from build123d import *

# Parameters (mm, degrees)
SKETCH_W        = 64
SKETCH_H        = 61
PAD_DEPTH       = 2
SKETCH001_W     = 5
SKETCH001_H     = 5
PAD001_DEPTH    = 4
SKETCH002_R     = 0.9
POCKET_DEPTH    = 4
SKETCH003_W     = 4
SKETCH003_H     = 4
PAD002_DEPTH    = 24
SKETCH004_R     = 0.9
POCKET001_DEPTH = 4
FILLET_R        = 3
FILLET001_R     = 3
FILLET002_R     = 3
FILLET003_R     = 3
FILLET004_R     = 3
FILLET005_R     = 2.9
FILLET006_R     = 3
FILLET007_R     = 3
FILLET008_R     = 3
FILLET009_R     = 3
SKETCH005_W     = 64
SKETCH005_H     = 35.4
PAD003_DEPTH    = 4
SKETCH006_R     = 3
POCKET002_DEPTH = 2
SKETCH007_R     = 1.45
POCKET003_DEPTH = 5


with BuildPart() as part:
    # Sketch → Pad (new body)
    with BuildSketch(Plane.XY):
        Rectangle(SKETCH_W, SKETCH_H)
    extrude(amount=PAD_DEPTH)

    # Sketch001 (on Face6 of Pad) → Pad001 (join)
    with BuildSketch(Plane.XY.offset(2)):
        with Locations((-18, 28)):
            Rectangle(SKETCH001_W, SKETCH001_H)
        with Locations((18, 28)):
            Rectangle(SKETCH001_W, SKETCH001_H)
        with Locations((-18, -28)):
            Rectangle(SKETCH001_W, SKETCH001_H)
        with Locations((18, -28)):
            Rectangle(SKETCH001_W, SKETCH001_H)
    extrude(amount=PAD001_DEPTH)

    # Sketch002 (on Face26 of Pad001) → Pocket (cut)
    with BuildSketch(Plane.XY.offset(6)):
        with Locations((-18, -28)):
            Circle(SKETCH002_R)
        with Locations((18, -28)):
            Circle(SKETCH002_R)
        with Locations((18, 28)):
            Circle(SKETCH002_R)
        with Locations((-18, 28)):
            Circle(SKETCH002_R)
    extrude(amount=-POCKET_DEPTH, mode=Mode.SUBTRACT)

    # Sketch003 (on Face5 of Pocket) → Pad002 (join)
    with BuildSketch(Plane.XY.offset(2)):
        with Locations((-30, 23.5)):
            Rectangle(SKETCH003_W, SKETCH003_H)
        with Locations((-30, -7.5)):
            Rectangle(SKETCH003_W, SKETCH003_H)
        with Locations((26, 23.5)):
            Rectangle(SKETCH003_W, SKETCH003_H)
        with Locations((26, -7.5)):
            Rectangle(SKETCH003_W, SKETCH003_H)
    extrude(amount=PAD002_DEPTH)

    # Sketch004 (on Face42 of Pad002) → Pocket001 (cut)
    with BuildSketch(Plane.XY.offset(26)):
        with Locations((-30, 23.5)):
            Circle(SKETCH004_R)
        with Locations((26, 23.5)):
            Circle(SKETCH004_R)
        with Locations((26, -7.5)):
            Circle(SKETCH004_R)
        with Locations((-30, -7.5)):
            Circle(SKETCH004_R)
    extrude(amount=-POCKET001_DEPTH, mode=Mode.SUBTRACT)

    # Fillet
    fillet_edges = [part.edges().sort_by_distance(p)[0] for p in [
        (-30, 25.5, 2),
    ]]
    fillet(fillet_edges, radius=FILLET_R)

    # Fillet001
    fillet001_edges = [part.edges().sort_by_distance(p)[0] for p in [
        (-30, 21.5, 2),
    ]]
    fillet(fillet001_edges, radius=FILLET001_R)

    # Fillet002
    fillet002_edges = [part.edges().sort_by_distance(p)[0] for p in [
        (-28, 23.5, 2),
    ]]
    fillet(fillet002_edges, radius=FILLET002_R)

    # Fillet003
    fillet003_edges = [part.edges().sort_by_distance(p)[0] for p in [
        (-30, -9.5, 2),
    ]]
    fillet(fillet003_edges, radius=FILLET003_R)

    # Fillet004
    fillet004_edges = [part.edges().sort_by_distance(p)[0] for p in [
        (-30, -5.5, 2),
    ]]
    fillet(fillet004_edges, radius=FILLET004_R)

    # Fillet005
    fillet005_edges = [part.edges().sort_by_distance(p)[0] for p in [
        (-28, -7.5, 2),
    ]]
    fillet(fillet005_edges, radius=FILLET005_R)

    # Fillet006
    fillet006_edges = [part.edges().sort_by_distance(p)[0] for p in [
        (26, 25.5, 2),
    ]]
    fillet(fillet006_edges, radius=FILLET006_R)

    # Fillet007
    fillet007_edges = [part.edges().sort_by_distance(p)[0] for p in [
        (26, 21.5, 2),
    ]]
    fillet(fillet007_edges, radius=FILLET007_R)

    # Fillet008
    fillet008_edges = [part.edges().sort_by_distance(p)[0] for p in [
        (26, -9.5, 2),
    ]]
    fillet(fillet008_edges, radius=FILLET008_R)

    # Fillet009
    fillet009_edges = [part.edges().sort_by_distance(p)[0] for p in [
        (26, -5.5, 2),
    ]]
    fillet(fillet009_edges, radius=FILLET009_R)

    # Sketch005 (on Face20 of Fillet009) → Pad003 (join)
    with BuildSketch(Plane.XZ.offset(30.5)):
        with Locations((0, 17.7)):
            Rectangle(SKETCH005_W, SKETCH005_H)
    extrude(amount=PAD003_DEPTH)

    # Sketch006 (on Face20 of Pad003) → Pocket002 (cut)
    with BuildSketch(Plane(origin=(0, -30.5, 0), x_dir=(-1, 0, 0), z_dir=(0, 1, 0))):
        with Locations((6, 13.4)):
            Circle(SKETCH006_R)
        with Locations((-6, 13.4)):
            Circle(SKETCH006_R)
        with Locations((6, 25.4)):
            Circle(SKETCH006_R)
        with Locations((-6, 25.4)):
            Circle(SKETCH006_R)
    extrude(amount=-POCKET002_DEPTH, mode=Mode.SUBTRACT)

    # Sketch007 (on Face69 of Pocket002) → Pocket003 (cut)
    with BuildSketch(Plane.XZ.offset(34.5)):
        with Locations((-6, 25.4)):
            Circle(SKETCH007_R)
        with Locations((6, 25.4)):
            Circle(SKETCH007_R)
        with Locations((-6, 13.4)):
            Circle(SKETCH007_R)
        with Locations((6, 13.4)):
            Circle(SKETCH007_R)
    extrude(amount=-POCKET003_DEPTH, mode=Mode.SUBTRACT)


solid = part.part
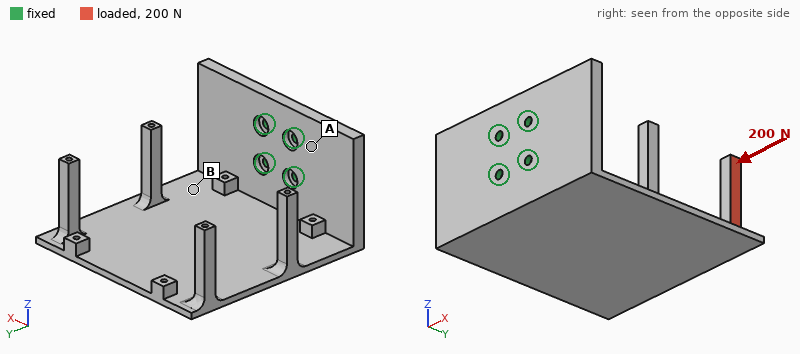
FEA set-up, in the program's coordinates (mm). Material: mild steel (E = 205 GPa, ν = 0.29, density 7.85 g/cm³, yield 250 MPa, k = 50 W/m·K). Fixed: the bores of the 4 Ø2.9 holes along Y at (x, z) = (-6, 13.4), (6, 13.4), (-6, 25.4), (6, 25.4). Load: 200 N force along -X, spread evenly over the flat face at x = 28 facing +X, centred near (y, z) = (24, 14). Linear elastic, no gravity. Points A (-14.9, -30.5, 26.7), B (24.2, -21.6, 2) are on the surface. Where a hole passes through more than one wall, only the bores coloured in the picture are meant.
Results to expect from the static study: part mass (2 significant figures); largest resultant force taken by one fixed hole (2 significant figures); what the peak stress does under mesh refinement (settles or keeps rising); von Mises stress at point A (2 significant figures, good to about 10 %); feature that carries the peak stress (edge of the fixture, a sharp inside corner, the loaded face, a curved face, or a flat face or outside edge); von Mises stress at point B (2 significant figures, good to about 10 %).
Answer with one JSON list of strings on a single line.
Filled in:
["150 g", "820 N", "keeps rising", "30 MPa", "edge of the fixture", "57 MPa"]
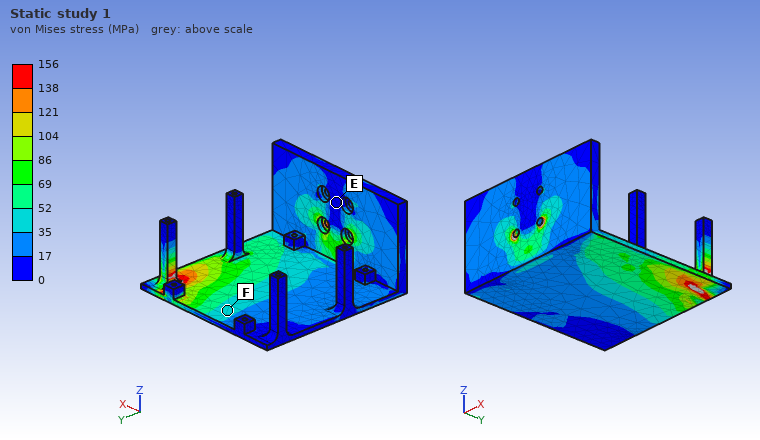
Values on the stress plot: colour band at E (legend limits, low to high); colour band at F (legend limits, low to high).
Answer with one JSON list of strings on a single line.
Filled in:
["0 to 17 MPa", "35 to 52 MPa"]
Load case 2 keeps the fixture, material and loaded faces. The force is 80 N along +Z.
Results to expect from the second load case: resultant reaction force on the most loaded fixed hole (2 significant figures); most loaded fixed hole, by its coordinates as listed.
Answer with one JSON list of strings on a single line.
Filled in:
["280 N", "(6, 25.4)"]
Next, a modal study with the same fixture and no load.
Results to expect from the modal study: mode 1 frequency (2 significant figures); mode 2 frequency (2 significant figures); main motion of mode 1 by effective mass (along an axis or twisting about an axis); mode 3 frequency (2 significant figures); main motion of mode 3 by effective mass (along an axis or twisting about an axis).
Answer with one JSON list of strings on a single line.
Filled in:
["380 Hz", "760 Hz", "along Z", "1100 Hz", "along X"]
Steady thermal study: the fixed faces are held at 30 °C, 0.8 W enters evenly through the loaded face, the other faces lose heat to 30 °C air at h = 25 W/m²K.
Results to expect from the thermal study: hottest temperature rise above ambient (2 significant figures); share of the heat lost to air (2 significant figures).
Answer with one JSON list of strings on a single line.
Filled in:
["17 K", "73 %"]
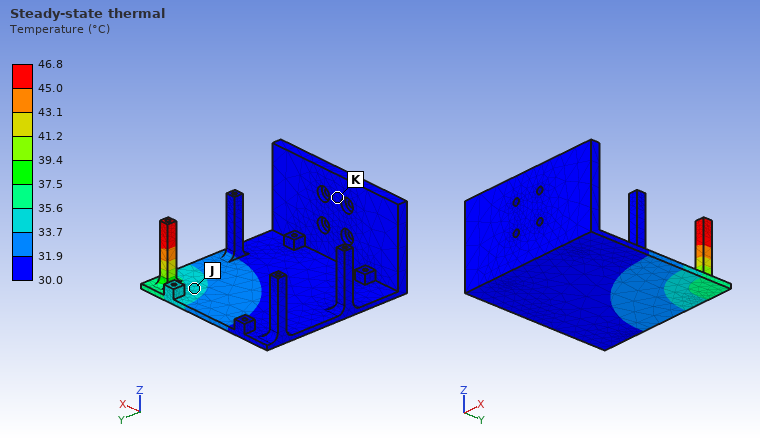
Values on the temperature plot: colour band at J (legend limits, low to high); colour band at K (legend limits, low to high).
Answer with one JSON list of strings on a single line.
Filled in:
["33.7 to 35.6 °C", "30.0 to 31.9 °C"]
